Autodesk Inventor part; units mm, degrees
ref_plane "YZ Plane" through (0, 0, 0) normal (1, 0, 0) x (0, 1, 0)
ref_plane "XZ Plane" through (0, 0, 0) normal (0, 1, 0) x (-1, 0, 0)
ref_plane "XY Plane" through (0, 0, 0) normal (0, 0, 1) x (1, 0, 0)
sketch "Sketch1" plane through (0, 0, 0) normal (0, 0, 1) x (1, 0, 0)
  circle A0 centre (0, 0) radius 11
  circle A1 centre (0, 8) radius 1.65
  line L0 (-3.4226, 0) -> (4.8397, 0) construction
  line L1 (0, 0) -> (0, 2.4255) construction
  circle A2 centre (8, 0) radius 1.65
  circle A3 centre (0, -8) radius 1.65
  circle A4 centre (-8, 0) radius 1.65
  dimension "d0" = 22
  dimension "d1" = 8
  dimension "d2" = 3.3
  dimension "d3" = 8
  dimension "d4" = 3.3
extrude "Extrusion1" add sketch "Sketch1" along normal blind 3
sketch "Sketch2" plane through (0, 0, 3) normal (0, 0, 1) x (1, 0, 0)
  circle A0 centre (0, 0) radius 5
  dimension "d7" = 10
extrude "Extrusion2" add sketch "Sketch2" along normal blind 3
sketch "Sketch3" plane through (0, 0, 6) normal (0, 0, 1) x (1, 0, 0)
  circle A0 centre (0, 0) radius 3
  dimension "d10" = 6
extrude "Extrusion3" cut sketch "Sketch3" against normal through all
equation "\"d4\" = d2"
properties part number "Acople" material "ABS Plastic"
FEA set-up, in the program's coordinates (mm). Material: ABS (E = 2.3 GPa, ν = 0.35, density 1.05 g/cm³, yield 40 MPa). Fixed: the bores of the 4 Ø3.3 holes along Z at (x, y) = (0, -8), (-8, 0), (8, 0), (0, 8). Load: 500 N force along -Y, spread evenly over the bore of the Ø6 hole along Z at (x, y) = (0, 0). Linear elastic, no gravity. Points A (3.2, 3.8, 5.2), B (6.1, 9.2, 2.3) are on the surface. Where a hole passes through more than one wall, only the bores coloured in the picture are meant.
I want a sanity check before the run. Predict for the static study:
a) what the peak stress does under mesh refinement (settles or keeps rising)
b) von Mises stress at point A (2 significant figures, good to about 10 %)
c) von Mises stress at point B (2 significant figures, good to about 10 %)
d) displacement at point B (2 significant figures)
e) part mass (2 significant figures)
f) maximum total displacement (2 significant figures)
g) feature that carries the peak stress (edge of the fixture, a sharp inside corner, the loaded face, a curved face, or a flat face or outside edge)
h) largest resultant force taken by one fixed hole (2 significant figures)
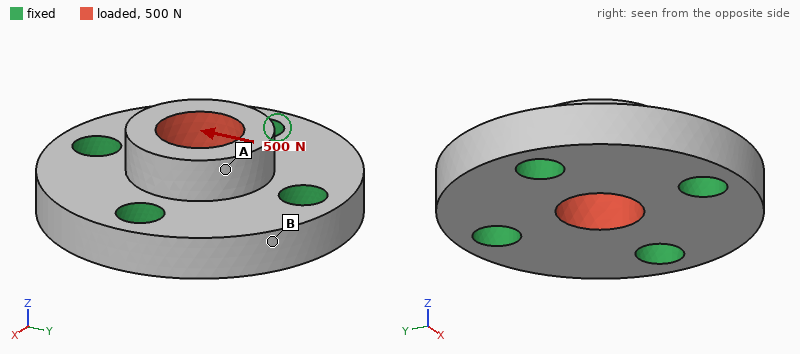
keeps rising
5.1 MPa
2.2 MPa
7.4 µm
1.2 g
49 µm
a sharp inside corner
170 N
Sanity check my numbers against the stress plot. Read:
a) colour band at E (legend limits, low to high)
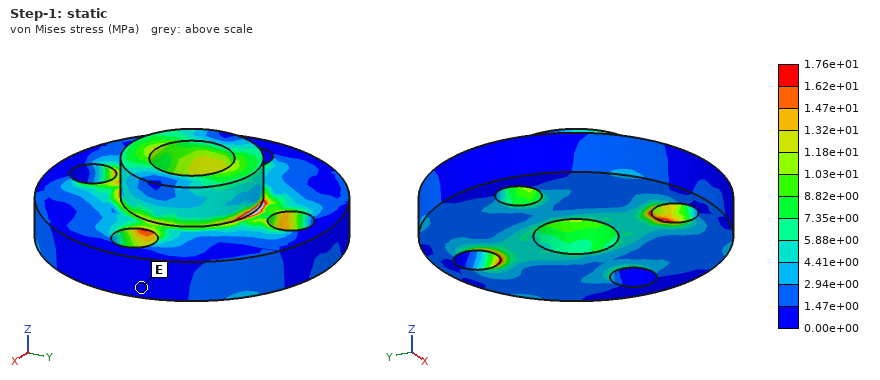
0.00e+00 to 1.47e+00 MPa
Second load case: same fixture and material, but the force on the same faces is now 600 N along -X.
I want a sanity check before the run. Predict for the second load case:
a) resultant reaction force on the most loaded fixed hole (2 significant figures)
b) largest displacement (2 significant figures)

200 N
58 µm
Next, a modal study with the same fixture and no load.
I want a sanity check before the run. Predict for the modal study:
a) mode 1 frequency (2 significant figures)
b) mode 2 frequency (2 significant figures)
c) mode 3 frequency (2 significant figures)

24 kHz
25 kHz
25 kHz
